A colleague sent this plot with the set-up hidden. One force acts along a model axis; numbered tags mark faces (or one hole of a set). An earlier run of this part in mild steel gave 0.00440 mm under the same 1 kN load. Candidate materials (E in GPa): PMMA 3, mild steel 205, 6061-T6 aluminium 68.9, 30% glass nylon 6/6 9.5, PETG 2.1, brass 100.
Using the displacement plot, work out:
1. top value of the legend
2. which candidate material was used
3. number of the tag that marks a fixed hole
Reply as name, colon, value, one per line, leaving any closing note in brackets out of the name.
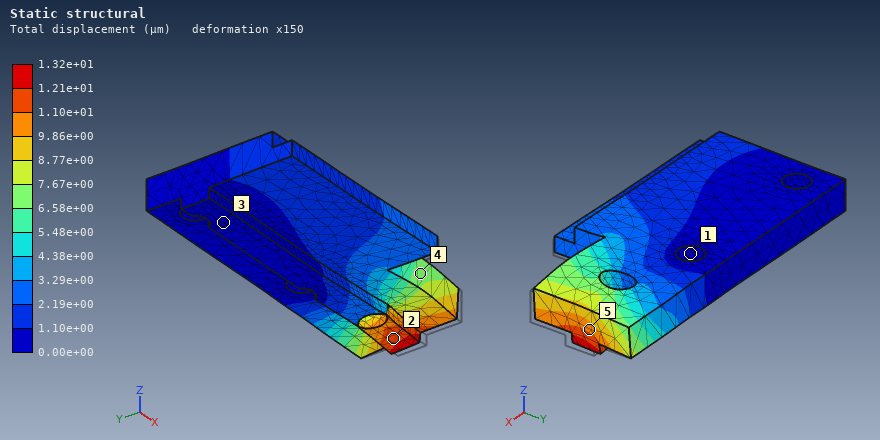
top value of the legend: 1.32e+01 µm
which candidate material was used: 6061-T6 aluminium
number of the tag that marks a fixed hole: 1
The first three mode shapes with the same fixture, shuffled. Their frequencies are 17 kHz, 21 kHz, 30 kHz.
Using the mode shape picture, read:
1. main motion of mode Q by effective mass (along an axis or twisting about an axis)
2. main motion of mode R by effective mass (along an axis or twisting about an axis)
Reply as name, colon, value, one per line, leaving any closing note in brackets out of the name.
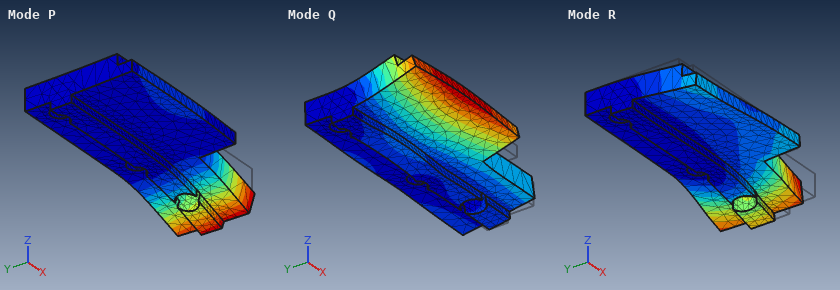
main motion of mode Q by effective mass: along Z
main motion of mode R by effective mass: along Y
